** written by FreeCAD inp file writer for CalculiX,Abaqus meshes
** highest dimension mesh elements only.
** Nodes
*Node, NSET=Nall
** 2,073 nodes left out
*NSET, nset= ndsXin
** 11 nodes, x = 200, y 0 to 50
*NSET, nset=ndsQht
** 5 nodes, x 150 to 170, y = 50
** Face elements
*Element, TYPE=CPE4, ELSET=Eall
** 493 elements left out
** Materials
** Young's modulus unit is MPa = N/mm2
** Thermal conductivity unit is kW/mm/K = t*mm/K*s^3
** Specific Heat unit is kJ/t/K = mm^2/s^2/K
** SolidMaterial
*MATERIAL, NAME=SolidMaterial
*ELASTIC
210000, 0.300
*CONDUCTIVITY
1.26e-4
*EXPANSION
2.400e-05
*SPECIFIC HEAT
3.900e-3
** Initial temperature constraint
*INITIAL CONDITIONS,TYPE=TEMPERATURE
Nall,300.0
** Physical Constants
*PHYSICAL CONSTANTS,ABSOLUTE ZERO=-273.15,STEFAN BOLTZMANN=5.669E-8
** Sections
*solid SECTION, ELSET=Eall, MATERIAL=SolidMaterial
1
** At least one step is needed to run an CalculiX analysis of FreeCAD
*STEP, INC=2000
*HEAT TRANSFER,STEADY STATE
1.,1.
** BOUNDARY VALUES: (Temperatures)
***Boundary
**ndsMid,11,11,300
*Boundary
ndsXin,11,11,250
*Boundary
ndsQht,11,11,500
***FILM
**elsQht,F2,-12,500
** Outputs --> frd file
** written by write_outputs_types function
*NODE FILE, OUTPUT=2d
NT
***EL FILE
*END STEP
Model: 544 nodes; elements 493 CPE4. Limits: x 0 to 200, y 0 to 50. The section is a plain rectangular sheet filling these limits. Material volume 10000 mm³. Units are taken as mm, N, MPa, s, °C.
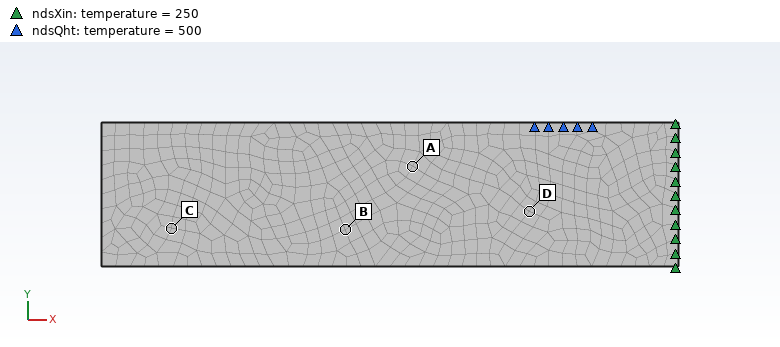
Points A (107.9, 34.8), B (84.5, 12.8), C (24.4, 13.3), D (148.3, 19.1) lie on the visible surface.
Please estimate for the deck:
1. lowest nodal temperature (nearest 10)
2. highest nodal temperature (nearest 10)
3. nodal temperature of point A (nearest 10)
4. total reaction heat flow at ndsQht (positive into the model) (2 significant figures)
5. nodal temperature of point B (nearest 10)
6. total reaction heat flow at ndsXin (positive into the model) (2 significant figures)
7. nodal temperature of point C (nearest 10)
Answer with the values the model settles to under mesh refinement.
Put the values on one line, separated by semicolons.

250 °C; 500 °C; 420 °C; 0.028 mW; 420 °C; -0.028 mW; 420 °C
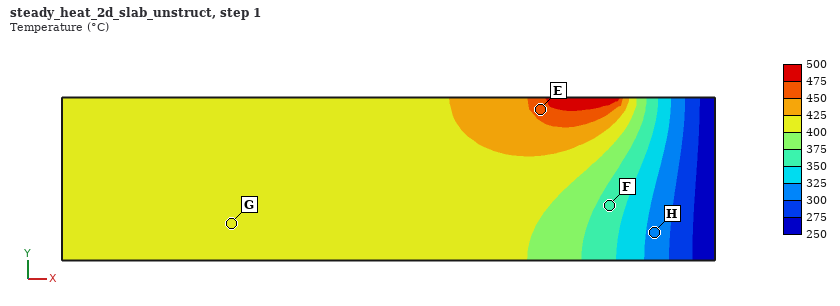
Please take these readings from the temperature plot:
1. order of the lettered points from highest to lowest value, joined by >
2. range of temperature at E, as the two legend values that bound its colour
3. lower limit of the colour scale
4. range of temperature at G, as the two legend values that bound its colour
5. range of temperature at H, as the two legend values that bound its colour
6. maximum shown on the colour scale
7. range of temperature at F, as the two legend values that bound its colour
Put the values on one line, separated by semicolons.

E > G > F > H; 450 to 475 °C; 250 °C; 400 to 425 °C; 300 to 325 °C; 500 °C; 350 to 375 °C
